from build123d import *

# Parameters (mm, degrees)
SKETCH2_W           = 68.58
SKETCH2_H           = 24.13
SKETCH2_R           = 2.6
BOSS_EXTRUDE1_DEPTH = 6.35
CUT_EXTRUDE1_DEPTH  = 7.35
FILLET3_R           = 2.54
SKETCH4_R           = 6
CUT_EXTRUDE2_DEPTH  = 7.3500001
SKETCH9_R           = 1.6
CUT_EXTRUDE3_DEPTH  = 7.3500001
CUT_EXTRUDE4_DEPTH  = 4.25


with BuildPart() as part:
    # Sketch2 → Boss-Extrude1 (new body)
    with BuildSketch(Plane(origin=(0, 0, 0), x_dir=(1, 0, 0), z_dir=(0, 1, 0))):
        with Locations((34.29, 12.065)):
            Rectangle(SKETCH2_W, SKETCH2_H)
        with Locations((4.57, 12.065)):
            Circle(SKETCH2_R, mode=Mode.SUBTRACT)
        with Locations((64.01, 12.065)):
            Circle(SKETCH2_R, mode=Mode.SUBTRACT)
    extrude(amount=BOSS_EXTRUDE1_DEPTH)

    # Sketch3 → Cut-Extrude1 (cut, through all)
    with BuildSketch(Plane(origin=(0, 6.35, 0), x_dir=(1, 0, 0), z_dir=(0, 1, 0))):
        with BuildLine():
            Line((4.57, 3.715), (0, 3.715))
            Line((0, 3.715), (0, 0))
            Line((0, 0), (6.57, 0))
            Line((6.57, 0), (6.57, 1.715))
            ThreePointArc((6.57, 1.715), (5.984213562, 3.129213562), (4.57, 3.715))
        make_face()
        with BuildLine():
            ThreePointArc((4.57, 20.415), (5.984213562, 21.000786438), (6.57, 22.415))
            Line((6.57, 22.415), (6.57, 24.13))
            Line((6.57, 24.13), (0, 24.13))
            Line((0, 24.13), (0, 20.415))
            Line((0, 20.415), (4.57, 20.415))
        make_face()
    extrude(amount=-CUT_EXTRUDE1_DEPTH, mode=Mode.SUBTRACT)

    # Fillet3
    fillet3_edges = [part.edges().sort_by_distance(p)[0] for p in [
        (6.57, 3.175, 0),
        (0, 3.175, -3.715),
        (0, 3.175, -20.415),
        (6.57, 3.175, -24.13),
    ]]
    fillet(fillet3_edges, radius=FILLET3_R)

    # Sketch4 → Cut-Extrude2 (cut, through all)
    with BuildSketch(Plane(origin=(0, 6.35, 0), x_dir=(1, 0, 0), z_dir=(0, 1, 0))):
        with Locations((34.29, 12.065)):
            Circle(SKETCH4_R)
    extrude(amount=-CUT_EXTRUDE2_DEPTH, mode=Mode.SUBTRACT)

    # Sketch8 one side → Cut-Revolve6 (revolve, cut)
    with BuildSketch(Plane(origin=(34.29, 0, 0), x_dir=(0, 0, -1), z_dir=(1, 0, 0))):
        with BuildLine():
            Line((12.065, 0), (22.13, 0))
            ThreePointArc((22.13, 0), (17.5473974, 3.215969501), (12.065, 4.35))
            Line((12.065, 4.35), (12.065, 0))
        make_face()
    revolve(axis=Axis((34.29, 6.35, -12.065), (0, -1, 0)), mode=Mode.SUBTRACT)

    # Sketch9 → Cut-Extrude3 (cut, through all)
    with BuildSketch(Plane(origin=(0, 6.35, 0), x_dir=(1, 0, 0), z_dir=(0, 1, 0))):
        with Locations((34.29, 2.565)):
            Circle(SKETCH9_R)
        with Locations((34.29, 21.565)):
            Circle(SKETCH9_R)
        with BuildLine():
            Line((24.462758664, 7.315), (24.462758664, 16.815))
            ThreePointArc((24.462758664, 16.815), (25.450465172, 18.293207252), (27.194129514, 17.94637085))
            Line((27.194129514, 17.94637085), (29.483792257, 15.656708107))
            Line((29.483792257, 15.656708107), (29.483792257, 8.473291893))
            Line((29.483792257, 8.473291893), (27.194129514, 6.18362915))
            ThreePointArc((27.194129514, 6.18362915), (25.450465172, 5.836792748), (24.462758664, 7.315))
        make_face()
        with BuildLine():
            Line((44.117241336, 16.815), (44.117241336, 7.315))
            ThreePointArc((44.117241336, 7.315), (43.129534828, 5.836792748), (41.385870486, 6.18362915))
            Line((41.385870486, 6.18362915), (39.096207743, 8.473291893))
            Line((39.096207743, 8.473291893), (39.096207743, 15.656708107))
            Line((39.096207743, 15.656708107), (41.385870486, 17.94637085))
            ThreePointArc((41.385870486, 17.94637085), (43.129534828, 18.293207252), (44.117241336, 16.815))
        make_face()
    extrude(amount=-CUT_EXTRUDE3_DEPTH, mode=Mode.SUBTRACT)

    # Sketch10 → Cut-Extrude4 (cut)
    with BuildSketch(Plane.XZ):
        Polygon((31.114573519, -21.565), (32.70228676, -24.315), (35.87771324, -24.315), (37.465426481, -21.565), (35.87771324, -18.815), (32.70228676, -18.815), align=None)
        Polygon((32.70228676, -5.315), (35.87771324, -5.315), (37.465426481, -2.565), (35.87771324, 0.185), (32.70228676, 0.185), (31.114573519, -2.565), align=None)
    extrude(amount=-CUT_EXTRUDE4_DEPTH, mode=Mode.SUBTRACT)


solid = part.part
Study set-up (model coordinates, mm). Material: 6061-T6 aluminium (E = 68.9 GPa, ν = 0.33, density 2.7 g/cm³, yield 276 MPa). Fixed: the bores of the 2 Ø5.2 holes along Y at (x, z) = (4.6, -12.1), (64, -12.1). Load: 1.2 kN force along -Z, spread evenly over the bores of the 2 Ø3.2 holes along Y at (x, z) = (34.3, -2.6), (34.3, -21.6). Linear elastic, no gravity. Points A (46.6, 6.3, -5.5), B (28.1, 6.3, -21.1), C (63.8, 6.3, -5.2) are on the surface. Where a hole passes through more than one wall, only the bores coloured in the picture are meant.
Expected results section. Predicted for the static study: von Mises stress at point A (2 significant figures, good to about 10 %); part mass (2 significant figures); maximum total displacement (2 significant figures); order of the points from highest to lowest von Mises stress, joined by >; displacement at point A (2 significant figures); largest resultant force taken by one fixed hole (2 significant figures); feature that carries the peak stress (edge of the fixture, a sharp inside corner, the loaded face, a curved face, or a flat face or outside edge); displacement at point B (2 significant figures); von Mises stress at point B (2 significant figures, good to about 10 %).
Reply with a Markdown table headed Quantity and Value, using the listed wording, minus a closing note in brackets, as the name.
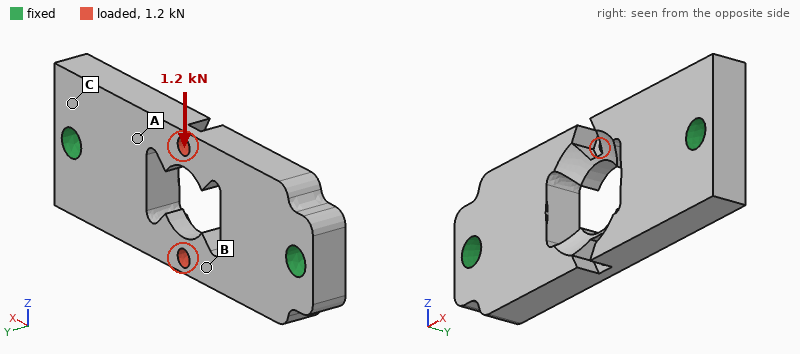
| Quantity | Value |
|---|---|
| von Mises stress at point A | 34 MPa |
| part mass | 22 g |
| maximum total displacement | 46 µm |
| order of the points from highest to lowest von Mises stress, joined by > | B > A > C |
| displacement at point A | 17 µm |
| largest resultant force taken by one fixed hole | 600 N |
| feature that carries the peak stress | the loaded face |
| displacement at point B | 31 µm |
| von Mises stress at point B | 58 MPa |
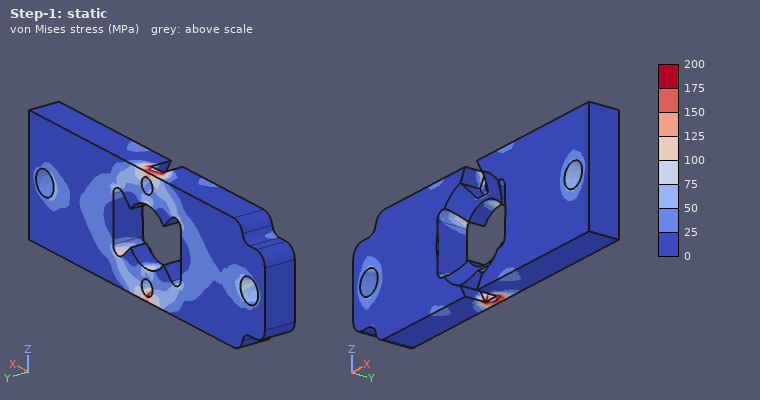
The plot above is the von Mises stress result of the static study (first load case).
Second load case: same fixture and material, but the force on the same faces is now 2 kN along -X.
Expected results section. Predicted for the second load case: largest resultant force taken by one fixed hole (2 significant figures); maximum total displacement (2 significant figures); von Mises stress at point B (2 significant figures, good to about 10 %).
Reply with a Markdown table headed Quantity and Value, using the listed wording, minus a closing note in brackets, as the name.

| Quantity | Value |
|---|---|
| largest resultant force taken by one fixed hole | 1.0 kN |
| maximum total displacement | 8.3 µm |
| von Mises stress at point B | 34 MPa |
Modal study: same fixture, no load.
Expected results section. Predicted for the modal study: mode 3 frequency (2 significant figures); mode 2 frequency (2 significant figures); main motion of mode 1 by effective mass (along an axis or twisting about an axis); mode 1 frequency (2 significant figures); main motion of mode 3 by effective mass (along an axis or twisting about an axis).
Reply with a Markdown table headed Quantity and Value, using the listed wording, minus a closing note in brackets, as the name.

| Quantity | Value |
|---|---|
| mode 3 frequency | 15 kHz |
| mode 2 frequency | 12 kHz |
| main motion of mode 1 by effective mass | along Y |
| mode 1 frequency | 8500 Hz |
| main motion of mode 3 by effective mass | along Z |
